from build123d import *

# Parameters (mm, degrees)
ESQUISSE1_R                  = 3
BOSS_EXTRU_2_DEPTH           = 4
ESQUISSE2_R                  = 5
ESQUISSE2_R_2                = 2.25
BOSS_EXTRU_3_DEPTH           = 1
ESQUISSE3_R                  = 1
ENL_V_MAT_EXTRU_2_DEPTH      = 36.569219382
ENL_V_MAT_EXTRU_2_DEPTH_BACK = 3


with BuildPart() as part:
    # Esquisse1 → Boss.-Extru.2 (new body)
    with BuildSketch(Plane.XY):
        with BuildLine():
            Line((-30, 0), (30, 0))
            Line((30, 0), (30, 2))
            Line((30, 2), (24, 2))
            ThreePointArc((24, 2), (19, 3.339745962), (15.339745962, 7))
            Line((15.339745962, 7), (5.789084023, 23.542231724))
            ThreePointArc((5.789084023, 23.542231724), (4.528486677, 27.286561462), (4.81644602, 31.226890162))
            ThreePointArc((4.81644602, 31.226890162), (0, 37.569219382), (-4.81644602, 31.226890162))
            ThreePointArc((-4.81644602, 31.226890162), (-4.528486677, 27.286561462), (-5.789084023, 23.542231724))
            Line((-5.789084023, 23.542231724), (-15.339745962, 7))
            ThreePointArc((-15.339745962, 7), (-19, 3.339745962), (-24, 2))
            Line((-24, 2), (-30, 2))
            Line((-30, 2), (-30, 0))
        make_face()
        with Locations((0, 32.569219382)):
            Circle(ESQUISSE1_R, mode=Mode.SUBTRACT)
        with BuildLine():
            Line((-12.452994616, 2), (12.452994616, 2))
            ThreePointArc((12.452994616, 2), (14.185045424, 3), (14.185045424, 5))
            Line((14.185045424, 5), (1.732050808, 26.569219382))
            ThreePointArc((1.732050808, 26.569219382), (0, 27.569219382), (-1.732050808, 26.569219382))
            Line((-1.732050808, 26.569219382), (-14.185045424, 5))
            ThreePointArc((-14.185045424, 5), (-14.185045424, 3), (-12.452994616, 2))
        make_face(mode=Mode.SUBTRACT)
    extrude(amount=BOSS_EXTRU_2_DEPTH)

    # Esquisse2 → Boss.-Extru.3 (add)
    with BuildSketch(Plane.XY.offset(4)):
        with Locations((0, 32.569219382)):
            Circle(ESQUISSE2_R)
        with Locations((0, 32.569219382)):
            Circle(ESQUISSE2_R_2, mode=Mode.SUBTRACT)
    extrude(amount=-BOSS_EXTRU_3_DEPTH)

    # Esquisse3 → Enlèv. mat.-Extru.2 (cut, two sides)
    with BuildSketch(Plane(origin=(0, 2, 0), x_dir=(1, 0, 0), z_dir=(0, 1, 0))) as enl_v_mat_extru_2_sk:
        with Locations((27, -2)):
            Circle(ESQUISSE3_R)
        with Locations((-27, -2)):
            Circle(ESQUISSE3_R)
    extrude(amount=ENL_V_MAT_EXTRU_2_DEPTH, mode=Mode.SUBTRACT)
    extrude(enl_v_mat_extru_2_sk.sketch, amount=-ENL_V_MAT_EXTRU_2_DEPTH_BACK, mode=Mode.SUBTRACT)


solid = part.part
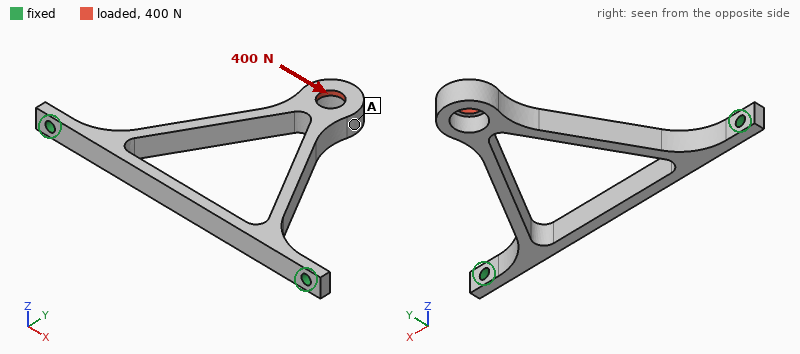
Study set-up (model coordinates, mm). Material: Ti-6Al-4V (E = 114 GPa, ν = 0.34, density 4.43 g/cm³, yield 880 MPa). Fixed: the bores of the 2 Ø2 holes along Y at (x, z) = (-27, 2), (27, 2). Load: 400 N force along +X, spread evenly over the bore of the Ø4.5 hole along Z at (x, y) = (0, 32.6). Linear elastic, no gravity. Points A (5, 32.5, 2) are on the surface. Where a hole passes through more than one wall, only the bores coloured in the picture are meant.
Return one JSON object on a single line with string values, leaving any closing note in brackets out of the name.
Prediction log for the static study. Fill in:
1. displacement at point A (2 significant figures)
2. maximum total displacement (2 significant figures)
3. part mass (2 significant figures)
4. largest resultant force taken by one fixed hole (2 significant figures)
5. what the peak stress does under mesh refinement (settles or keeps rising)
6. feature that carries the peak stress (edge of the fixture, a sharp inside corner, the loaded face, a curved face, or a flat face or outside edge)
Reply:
{"displacement at point A": "0.17 mm", "maximum total displacement": "0.24 mm", "part mass": "5.6 g", "largest resultant force taken by one fixed hole": "350 N", "what the peak stress does under mesh refinement": "keeps rising", "feature that carries the peak stress": "edge of the fixture"}
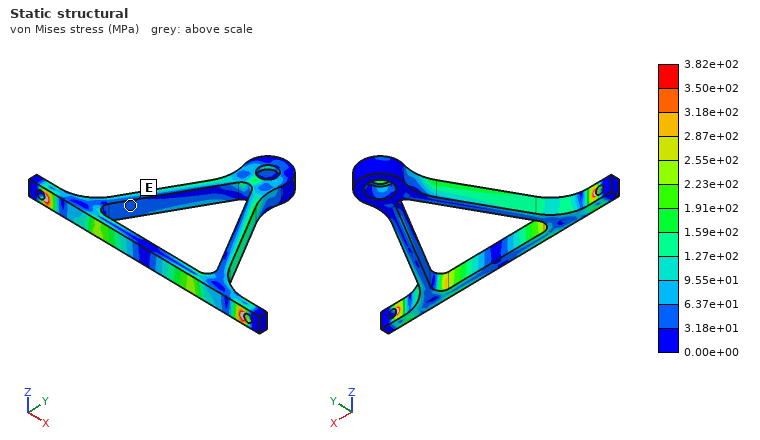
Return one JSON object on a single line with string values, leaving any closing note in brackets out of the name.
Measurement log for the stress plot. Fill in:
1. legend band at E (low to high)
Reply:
{"legend band at E": "3.18e+01 to 6.37e+01 MPa"}
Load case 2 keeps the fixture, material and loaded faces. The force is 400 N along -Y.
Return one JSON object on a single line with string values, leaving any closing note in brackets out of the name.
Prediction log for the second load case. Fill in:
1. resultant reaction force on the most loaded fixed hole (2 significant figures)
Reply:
{"resultant reaction force on the most loaded fixed hole": "240 N"}
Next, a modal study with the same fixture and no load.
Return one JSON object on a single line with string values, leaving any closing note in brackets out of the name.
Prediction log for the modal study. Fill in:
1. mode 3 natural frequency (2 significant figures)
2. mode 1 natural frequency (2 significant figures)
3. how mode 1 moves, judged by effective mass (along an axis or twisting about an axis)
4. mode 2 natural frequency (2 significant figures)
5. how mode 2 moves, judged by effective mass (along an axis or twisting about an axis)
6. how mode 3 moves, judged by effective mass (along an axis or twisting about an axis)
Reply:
{"mode 3 natural frequency": "5000 Hz", "mode 1 natural frequency": "1100 Hz", "how mode 1 moves, judged by effective mass": "along Z", "mode 2 natural frequency": "3800 Hz", "how mode 2 moves, judged by effective mass": "along Y", "how mode 3 moves, judged by effective mass": "twisting about Z"}
